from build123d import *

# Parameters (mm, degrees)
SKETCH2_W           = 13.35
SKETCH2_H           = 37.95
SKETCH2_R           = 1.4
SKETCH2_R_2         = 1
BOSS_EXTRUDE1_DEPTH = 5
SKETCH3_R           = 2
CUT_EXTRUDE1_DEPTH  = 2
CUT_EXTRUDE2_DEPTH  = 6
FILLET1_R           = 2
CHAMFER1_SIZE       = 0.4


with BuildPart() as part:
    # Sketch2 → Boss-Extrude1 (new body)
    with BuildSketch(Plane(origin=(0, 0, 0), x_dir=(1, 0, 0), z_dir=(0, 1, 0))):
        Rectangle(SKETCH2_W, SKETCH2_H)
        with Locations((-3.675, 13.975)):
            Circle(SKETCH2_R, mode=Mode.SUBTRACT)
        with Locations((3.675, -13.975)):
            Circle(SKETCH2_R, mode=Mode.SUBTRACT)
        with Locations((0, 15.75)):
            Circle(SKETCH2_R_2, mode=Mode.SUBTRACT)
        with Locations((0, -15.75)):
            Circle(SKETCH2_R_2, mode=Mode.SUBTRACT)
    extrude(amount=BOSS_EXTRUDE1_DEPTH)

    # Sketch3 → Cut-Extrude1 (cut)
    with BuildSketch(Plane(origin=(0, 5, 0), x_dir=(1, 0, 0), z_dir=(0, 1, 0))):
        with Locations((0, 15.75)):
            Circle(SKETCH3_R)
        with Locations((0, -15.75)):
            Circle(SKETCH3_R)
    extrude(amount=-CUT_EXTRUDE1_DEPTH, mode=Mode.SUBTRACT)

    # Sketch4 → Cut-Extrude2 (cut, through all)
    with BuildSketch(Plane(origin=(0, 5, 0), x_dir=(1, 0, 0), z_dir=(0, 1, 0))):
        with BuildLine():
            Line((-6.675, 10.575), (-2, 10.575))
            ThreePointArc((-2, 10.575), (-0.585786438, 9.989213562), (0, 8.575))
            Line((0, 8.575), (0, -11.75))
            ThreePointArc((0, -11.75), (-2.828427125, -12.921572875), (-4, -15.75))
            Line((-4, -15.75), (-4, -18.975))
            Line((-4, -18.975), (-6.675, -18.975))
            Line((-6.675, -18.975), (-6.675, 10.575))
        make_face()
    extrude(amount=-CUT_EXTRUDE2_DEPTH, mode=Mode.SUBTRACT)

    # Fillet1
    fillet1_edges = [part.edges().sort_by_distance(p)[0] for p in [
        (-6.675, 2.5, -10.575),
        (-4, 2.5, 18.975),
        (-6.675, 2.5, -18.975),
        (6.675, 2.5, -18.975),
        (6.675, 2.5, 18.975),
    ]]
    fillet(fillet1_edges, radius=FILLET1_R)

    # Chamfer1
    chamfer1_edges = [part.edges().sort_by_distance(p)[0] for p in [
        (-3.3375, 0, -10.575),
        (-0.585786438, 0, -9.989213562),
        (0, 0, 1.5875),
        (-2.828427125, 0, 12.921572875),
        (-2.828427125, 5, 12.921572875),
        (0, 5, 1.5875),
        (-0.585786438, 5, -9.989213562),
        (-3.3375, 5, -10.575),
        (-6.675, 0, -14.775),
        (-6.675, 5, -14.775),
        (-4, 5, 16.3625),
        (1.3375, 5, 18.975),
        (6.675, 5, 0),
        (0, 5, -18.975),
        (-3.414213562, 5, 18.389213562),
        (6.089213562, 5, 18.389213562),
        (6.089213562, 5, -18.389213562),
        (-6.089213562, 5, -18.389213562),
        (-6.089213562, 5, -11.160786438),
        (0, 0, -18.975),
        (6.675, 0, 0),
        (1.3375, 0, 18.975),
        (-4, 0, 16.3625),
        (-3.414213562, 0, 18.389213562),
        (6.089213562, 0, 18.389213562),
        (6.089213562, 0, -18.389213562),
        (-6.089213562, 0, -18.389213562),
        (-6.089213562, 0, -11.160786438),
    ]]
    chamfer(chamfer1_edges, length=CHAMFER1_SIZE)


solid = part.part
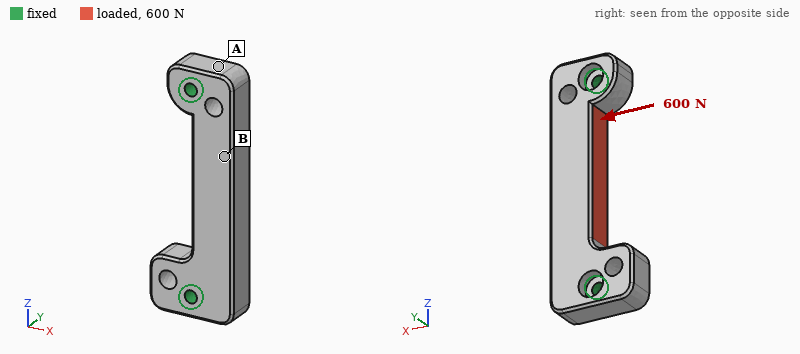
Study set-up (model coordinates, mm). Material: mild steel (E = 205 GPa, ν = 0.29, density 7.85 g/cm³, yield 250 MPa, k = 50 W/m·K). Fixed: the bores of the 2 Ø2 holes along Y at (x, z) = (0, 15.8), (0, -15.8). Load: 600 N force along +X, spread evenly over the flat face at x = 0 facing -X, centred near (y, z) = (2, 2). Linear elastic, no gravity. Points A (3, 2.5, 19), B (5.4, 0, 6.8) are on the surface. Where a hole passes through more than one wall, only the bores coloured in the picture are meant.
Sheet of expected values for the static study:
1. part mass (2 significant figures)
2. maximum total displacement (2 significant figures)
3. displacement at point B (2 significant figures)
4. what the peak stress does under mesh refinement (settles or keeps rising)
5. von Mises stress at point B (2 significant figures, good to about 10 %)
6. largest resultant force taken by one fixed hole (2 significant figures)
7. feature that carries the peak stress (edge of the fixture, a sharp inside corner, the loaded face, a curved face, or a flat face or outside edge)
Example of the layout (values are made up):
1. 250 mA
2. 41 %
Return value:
1. 12 g
2. 5.5 µm
3. 3.8 µm
4. keeps rising
5. 27 MPa
6. 450 N
7. edge of the fixture
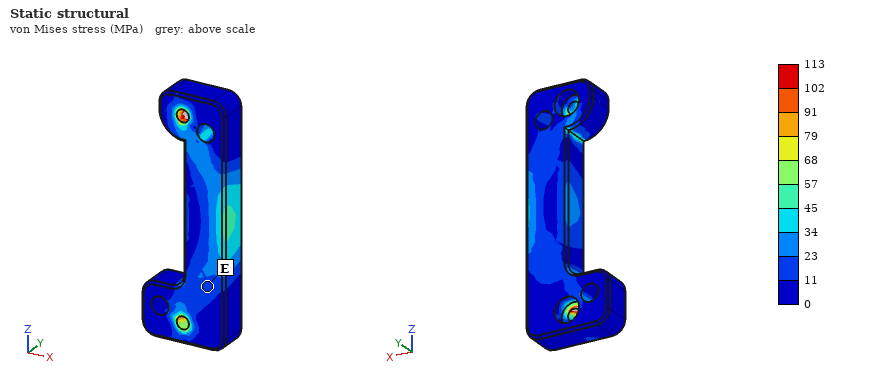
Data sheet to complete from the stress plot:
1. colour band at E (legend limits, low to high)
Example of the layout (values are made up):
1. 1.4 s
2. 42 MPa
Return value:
1. 11 to 23 MPa
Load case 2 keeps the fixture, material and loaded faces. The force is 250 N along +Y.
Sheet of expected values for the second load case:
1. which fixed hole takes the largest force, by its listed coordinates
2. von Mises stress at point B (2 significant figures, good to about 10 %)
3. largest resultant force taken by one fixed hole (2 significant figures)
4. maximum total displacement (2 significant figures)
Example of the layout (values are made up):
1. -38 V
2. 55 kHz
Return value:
1. (0, 15.8)
2. 15 MPa
3. 150 N
4. 5.0 µm
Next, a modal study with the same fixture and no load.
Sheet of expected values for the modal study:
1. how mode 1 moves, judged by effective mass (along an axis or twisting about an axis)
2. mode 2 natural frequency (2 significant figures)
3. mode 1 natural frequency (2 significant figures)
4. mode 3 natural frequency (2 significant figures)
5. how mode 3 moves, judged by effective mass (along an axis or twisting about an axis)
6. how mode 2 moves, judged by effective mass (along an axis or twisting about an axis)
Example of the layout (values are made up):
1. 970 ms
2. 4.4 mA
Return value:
1. along Y
2. 25 kHz
3. 16 kHz
4. 32 kHz
5. twisting about Z
6. along X
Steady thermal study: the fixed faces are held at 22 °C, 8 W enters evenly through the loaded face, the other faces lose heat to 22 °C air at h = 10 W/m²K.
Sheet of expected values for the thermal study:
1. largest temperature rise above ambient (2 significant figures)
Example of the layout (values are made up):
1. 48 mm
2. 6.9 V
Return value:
1. 33 K
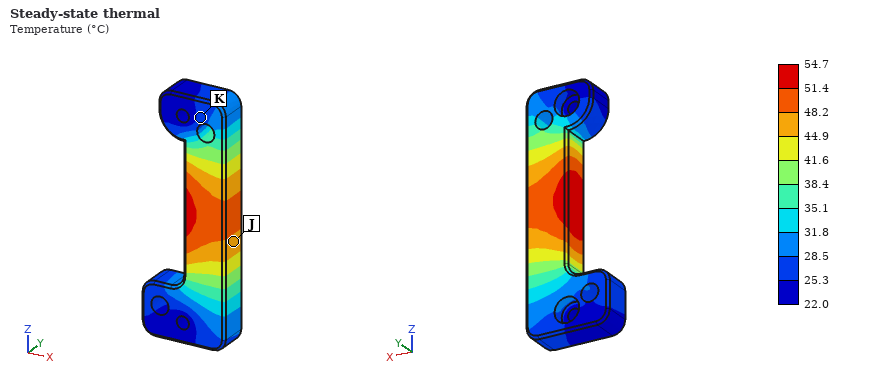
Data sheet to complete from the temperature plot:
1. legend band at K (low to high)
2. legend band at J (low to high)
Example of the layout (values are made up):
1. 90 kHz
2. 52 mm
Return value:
1. 25.3 to 28.5 °C
2. 44.9 to 48.2 °C
